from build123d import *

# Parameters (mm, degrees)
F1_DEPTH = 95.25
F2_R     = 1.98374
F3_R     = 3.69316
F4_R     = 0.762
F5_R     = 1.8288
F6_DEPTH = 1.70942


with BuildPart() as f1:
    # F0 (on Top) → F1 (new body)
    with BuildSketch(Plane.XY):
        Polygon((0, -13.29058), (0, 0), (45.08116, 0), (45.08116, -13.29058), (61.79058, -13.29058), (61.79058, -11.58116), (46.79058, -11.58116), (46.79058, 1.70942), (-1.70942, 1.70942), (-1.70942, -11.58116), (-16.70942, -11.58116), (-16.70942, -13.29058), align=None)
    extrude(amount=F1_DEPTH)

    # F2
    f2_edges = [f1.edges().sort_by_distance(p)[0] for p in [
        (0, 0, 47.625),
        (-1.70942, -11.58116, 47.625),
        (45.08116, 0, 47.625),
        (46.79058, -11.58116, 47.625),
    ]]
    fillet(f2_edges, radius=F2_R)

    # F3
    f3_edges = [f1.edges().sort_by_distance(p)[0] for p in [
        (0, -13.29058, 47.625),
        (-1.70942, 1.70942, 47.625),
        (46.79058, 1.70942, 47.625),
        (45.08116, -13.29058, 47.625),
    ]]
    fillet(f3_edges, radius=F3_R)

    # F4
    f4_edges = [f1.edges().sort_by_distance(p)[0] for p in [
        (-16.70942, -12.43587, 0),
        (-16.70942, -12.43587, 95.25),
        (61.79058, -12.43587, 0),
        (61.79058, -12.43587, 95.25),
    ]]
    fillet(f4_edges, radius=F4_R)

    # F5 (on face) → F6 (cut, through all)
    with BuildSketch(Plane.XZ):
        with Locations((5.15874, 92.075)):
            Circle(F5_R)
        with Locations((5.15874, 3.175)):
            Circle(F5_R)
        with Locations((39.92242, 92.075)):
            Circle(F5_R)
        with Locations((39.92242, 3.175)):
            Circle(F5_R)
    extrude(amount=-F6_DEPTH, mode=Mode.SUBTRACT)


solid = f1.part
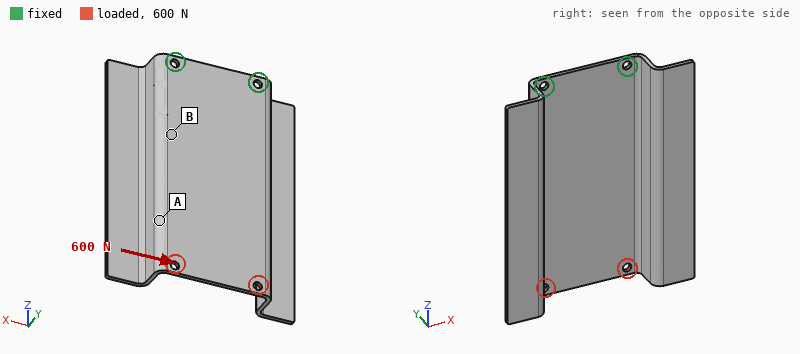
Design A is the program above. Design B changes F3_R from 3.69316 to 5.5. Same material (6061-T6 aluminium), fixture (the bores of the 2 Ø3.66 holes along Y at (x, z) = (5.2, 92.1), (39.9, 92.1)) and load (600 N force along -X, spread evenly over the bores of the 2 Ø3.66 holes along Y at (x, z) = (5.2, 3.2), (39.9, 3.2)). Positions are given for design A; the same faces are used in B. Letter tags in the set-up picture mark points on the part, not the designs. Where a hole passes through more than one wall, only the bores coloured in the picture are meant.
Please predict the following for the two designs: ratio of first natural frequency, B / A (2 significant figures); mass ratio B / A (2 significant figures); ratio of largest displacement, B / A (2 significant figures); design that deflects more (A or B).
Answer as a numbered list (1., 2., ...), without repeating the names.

1. 0.97
2. 0.92
3. 1.2
4. B
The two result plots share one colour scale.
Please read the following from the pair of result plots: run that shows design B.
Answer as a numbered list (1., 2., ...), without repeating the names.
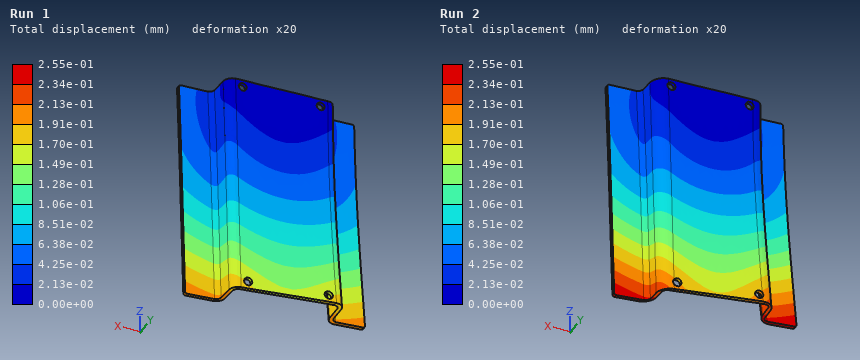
1. Run 2
